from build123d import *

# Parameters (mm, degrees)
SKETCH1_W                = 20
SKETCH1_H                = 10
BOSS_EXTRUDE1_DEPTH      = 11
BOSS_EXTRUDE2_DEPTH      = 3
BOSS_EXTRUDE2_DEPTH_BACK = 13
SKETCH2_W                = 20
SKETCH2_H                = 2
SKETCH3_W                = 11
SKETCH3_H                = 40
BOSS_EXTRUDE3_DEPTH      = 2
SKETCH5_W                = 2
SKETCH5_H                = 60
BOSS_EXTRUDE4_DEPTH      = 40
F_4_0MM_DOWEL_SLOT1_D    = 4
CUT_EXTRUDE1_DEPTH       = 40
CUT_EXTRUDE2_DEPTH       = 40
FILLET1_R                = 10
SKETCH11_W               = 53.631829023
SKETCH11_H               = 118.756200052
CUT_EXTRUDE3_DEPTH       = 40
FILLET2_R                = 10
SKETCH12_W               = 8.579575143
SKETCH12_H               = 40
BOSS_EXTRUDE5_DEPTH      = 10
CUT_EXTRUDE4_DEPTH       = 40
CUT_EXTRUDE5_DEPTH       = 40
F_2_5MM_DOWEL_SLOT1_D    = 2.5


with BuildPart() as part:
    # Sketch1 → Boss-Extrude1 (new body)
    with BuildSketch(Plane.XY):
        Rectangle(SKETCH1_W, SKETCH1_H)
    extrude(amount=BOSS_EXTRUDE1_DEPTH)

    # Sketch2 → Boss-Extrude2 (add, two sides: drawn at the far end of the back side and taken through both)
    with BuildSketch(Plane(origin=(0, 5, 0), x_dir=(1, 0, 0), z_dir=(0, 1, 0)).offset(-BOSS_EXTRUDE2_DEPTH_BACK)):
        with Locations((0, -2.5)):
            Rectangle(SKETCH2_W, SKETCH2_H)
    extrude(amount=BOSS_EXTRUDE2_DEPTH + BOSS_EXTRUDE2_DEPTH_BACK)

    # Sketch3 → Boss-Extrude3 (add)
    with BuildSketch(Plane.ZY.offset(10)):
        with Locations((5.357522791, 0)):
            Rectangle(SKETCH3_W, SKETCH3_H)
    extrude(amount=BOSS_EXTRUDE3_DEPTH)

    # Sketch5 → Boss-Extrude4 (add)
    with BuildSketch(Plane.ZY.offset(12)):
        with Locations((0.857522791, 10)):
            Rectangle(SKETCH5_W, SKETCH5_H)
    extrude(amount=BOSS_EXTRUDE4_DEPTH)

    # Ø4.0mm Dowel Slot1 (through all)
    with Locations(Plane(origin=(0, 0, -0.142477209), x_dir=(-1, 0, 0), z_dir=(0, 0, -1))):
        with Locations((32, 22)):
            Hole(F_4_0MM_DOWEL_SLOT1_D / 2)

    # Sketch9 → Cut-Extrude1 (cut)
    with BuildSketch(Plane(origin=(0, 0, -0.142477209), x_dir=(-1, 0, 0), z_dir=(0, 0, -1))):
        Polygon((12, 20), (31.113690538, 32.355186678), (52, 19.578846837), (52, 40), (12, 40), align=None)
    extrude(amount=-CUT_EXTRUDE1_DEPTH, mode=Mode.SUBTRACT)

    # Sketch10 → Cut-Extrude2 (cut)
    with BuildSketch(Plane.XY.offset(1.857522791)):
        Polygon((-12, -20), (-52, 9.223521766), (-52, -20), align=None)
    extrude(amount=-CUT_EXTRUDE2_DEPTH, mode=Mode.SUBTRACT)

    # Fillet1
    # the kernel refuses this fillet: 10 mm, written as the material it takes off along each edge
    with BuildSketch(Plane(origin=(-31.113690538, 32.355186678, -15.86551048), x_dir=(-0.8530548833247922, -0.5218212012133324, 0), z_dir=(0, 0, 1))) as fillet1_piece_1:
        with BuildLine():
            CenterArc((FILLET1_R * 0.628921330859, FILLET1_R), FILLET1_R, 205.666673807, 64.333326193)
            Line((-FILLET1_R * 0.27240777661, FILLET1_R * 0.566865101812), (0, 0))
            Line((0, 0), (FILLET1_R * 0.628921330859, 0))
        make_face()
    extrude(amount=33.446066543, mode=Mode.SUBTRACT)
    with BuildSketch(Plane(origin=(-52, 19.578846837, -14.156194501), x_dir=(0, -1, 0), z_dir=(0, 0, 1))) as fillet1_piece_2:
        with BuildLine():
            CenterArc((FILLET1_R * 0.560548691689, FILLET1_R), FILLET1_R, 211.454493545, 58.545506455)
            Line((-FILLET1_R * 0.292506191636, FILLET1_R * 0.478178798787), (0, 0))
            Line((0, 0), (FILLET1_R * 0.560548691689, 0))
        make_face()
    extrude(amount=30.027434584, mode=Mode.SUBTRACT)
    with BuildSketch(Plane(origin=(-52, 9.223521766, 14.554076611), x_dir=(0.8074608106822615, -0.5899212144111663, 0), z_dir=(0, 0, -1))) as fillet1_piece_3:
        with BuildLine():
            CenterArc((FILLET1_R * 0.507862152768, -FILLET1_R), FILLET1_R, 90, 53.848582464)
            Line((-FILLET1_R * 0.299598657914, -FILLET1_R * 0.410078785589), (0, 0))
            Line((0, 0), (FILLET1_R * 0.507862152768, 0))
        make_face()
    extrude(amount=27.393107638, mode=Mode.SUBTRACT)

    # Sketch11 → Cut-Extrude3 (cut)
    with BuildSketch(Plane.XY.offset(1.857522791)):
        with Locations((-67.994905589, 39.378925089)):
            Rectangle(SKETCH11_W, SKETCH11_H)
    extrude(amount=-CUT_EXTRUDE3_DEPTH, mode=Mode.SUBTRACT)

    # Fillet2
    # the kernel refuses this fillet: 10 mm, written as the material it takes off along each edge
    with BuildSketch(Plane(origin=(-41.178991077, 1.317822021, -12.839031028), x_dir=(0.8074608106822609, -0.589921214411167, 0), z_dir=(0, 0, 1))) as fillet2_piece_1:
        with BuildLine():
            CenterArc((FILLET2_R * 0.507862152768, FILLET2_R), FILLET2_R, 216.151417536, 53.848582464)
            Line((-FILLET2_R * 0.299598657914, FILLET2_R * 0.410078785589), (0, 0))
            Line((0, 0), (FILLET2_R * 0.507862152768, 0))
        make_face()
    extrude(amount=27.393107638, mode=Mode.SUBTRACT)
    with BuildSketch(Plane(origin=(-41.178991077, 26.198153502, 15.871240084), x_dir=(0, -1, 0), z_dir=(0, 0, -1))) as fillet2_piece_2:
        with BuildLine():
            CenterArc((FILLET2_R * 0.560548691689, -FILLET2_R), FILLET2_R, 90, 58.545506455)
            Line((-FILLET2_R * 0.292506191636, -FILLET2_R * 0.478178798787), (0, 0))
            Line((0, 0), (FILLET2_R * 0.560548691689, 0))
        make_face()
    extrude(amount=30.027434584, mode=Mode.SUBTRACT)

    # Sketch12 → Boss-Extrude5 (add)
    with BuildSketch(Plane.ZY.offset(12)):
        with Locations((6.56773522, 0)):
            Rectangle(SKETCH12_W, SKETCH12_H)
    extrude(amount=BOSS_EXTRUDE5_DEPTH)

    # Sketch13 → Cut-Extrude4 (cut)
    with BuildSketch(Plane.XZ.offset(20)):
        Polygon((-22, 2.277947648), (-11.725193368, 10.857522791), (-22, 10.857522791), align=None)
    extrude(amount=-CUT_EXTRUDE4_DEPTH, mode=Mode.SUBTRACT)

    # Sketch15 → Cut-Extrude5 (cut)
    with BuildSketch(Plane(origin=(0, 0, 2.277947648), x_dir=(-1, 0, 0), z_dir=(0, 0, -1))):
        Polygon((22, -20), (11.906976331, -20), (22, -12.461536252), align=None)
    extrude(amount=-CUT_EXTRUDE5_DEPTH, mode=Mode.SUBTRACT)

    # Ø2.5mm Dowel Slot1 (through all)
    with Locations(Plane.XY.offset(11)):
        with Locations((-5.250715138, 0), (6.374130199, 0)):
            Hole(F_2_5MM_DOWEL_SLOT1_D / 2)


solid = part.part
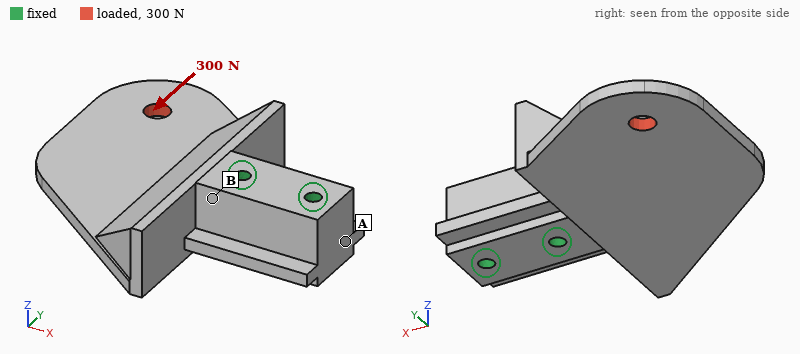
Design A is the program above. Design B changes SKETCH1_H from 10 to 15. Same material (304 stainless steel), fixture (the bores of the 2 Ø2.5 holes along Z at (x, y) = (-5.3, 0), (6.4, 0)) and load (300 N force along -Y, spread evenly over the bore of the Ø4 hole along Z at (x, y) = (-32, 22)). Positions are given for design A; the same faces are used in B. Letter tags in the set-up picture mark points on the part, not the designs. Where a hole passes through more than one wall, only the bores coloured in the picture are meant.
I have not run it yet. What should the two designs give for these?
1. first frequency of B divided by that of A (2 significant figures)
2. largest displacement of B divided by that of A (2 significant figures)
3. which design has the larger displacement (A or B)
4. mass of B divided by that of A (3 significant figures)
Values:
1.0
0.75
A
1.13
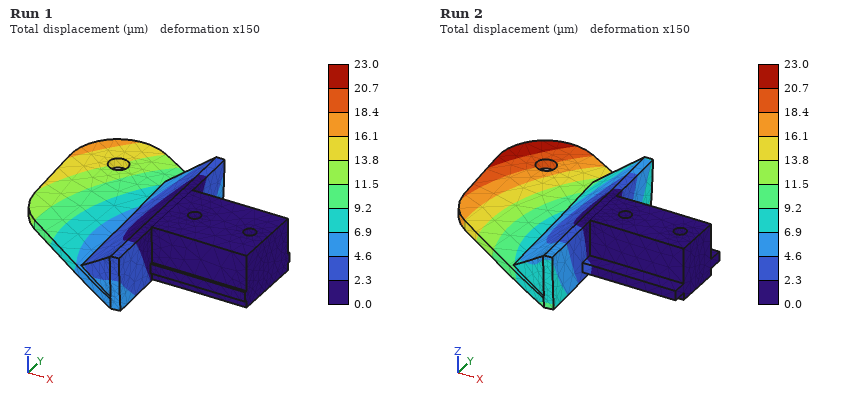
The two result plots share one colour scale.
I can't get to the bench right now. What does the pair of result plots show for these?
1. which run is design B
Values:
Run 1
